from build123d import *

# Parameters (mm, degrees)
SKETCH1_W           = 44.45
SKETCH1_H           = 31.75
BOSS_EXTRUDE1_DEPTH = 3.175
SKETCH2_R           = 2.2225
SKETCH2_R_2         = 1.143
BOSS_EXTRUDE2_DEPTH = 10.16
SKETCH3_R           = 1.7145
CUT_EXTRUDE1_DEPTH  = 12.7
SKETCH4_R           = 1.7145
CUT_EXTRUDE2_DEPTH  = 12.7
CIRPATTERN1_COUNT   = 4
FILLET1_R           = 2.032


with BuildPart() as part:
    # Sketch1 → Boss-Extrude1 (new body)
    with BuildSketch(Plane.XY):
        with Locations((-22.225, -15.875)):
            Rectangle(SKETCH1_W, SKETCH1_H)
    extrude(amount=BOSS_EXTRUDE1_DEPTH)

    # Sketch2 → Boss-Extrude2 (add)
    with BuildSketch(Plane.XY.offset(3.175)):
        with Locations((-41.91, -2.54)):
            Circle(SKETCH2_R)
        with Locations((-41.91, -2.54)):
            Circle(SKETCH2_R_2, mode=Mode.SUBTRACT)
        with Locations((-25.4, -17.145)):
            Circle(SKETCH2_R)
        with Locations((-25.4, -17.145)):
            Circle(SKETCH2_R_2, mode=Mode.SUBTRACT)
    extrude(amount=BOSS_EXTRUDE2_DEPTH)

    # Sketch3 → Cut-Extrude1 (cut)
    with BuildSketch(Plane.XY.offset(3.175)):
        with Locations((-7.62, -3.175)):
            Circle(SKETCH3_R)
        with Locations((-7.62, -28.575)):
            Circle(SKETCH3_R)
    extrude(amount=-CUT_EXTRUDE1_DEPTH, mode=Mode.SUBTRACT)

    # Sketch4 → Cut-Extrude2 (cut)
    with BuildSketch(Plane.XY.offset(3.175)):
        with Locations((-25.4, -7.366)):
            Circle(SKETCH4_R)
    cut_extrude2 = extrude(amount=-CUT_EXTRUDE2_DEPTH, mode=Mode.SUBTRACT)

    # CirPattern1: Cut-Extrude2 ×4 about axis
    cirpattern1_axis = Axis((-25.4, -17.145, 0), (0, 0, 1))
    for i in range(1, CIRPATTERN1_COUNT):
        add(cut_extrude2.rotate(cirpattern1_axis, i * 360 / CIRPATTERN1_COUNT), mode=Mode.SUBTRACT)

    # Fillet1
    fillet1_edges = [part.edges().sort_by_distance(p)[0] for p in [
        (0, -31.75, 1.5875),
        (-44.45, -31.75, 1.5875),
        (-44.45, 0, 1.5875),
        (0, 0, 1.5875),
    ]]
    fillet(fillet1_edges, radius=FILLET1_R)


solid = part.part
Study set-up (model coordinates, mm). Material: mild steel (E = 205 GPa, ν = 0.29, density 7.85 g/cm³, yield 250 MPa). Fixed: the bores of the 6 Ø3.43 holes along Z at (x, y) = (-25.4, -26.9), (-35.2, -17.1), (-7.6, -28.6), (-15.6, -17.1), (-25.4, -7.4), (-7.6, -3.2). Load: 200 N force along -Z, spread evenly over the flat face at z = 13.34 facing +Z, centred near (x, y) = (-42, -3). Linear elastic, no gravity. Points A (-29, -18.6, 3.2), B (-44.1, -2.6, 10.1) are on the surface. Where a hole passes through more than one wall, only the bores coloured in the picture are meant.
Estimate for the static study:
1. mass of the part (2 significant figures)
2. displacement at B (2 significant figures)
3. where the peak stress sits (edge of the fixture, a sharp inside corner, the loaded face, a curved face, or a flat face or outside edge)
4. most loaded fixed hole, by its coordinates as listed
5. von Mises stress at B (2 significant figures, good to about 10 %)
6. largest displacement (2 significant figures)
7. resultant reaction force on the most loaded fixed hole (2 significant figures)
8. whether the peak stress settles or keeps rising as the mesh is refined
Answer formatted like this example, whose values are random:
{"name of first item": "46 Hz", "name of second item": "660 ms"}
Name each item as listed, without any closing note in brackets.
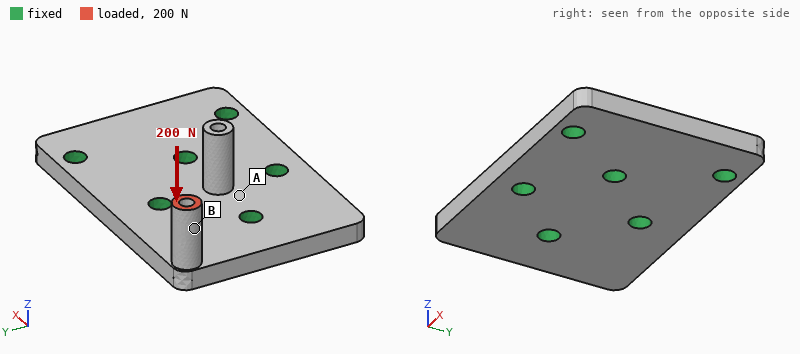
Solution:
{"mass of the part": "36 g", "displacement at B": "29 µm", "where the peak stress sits": "edge of the fixture", "most loaded fixed hole, by its coordinates as listed": "(-35.2, -17.1)", "von Mises stress at B": "18 MPa", "largest displacement": "35 µm", "resultant reaction force on the most loaded fixed hole": "140 N", "whether the peak stress settles or keeps rising as the mesh is refined": "keeps rising"}
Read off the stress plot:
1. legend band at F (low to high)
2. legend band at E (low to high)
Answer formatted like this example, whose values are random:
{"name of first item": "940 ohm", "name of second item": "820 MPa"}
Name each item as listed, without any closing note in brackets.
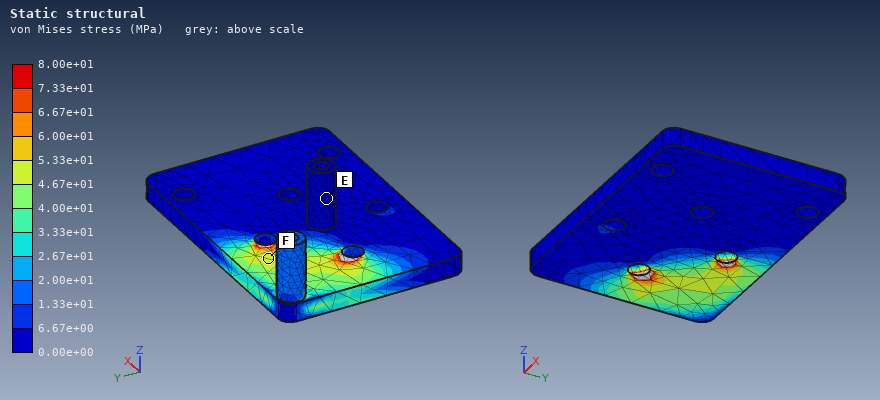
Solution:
{"legend band at F": "4.67e+01 to 5.33e+01 MPa", "legend band at E": "0.00e+00 to 6.67e+00 MPa"}
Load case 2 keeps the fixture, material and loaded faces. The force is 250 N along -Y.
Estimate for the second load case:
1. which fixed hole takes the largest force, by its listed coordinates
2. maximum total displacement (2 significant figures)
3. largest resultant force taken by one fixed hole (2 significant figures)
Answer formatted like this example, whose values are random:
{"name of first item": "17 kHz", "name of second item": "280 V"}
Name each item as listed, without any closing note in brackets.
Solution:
{"which fixed hole takes the largest force, by its listed coordinates": "(-35.2, -17.1)", "maximum total displacement": "91 µm", "largest resultant force taken by one fixed hole": "280 N"}
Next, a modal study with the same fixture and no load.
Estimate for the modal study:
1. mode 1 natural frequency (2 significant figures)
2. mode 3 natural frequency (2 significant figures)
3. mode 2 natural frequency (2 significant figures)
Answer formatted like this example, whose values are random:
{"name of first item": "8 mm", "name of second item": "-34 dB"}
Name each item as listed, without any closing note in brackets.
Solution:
{"mode 1 natural frequency": "9500 Hz", "mode 3 natural frequency": "17 kHz", "mode 2 natural frequency": "17 kHz"}
